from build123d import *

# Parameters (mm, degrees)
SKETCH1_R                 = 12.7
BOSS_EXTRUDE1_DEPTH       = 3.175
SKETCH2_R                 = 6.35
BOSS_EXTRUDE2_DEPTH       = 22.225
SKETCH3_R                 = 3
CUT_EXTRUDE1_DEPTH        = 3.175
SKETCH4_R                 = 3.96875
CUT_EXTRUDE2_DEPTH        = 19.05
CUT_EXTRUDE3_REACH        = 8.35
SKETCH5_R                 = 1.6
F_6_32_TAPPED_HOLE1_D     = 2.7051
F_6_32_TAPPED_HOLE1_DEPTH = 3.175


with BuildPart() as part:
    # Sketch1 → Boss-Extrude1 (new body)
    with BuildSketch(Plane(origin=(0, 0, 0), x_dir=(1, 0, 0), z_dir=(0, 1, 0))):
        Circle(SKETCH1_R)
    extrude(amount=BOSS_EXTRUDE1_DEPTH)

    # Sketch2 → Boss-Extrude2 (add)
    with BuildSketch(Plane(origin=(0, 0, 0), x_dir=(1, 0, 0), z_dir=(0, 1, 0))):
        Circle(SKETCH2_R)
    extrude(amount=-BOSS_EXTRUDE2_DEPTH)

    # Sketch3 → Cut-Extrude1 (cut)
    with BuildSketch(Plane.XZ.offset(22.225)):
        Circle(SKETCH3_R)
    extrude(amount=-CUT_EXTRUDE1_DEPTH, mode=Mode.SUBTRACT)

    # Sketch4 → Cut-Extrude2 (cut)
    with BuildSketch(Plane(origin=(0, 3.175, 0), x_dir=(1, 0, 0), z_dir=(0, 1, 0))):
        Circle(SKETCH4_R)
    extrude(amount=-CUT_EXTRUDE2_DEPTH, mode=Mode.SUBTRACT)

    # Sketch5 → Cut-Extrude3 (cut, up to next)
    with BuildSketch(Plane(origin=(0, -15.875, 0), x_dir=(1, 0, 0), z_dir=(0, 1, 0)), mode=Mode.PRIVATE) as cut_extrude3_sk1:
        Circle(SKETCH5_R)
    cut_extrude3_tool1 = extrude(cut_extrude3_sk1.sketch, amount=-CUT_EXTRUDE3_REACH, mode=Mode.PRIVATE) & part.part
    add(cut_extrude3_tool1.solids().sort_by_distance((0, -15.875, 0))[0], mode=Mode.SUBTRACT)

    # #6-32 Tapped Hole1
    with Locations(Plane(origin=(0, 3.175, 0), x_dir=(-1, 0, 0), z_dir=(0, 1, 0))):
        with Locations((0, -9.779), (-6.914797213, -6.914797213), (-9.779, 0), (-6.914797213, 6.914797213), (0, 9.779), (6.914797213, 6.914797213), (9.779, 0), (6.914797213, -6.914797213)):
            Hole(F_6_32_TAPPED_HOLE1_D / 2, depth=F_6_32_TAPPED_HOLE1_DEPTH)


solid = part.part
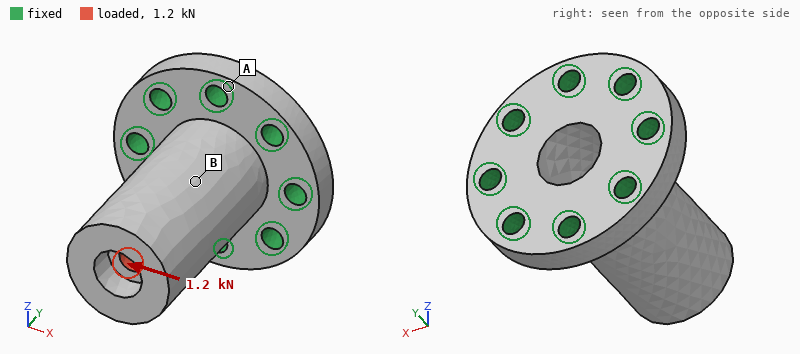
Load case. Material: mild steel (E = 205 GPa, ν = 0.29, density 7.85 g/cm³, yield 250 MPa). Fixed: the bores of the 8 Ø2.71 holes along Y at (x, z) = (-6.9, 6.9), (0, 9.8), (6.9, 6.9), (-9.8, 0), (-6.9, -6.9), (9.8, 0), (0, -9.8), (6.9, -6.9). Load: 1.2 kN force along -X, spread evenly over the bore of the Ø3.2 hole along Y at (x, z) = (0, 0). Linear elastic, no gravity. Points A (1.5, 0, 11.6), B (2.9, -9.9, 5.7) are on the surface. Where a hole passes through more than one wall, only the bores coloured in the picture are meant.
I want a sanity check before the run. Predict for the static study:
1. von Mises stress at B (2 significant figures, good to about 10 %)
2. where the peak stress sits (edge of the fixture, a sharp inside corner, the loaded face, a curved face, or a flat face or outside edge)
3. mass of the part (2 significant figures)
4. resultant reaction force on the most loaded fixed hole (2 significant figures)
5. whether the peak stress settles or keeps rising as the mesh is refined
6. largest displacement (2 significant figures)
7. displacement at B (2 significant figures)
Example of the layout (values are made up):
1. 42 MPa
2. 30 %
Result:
1. 45 MPa
2. edge of the fixture
3. 25 g
4. 810 N
5. keeps rising
6. 32 µm
7. 13 µm
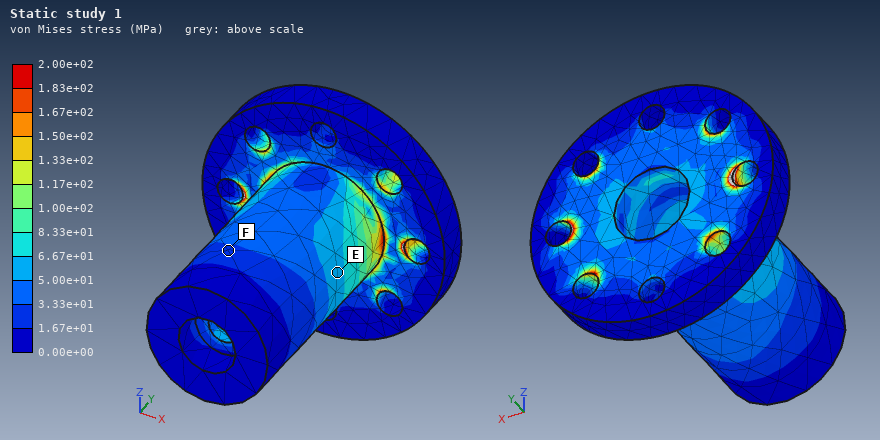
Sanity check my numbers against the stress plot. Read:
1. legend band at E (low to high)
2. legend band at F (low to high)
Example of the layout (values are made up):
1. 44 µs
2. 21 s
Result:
1. 5.00e+01 to 6.67e+01 MPa
2. 1.67e+01 to 3.33e+01 MPa
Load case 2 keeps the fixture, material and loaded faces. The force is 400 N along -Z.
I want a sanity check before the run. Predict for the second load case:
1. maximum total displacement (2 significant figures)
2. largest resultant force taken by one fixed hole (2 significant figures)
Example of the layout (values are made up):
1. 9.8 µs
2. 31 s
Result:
1. 11 µm
2. 270 N
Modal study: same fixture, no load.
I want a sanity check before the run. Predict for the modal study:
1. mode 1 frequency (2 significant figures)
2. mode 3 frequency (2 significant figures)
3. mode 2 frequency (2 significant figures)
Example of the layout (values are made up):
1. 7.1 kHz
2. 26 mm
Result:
1. 12 kHz
2. 32 kHz
3. 12 kHz
